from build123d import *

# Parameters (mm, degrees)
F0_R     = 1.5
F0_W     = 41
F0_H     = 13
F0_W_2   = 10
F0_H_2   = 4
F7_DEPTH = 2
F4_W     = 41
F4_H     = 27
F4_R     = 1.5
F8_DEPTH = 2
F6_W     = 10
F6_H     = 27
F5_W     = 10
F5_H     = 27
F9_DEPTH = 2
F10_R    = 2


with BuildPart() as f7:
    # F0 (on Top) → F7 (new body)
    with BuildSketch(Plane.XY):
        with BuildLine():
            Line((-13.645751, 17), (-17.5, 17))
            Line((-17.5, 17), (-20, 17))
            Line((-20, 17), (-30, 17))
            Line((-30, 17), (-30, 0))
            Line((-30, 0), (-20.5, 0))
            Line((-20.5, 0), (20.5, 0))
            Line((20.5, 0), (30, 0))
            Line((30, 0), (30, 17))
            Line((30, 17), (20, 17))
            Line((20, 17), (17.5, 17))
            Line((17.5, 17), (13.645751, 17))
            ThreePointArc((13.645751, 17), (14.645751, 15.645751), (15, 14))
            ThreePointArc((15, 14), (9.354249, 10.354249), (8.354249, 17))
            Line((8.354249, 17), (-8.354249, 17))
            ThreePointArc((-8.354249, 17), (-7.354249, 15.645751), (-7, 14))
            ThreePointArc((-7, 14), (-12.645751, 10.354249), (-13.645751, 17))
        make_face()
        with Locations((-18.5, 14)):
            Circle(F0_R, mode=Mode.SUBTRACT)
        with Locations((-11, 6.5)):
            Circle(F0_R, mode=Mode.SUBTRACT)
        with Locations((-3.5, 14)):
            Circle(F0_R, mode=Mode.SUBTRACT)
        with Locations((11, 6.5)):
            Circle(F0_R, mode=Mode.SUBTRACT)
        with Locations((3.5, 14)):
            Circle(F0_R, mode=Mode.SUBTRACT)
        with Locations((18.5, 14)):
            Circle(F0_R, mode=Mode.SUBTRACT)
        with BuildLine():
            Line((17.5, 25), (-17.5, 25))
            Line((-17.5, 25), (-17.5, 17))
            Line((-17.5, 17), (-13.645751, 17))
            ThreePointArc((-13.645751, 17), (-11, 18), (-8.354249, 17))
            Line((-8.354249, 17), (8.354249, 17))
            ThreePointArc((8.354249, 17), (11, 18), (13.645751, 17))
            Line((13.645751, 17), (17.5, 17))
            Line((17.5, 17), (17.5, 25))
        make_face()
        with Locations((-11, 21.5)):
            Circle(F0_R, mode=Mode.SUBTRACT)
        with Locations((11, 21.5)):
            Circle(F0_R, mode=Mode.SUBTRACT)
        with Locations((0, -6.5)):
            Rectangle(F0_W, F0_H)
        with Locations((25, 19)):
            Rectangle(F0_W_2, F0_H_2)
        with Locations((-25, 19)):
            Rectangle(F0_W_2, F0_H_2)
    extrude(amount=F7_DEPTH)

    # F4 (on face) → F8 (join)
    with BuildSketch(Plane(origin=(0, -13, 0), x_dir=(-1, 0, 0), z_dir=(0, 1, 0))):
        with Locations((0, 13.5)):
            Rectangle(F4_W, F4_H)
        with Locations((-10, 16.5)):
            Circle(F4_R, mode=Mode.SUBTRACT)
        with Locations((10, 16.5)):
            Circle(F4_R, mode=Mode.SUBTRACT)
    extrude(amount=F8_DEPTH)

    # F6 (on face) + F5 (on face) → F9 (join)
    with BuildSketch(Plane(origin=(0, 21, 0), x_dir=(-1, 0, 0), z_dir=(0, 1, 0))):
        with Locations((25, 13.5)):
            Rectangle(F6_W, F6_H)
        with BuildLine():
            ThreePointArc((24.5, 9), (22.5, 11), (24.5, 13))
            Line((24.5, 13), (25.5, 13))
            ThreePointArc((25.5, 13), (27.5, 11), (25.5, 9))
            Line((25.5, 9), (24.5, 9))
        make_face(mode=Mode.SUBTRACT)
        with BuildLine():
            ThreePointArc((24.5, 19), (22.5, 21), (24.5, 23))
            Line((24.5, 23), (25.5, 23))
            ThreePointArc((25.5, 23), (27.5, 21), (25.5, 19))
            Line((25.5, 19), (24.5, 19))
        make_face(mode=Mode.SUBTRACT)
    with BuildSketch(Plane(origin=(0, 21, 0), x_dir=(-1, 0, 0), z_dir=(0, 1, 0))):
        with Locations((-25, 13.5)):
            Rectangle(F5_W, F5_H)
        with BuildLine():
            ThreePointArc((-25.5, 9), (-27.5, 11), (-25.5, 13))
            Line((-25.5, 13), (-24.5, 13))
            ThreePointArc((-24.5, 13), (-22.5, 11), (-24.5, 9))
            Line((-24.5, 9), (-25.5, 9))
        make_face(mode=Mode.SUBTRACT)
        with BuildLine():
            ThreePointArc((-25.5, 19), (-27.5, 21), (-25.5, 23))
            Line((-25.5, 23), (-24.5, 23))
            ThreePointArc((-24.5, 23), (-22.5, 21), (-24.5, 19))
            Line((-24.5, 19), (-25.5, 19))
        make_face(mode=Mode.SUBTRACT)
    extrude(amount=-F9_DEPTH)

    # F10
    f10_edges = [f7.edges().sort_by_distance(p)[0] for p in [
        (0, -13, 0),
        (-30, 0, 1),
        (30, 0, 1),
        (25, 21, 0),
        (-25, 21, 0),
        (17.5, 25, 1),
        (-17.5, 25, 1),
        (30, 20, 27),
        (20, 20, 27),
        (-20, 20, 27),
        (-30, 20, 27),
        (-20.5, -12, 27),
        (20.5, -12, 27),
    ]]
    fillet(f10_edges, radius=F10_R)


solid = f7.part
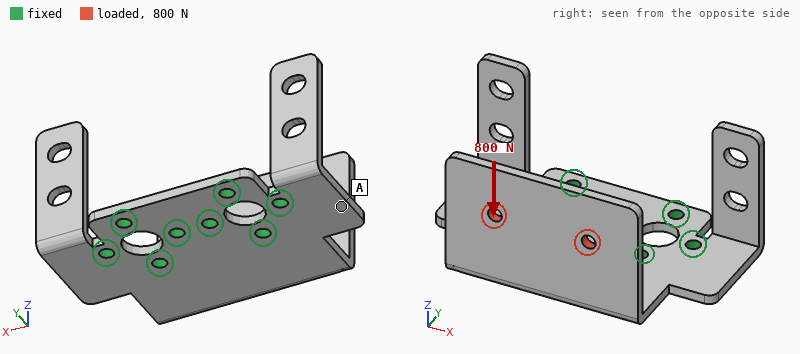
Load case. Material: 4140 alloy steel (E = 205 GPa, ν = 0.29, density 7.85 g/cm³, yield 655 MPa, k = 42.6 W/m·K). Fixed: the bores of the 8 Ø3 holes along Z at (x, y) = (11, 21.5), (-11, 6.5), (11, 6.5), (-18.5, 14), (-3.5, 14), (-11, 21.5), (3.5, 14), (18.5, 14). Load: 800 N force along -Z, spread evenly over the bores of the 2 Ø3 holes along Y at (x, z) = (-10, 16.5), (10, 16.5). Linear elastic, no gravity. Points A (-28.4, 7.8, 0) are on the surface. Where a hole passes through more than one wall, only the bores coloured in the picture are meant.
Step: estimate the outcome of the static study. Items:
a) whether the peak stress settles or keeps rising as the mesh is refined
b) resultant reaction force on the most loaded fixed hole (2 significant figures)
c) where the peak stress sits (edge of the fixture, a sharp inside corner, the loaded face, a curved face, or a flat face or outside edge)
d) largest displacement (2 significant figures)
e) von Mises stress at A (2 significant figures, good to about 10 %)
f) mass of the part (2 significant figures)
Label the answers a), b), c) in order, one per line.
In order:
a) keeps rising
b) 730 N
c) edge of the fixture
d) 0.66 mm
e) 68 MPa
f) 50 g
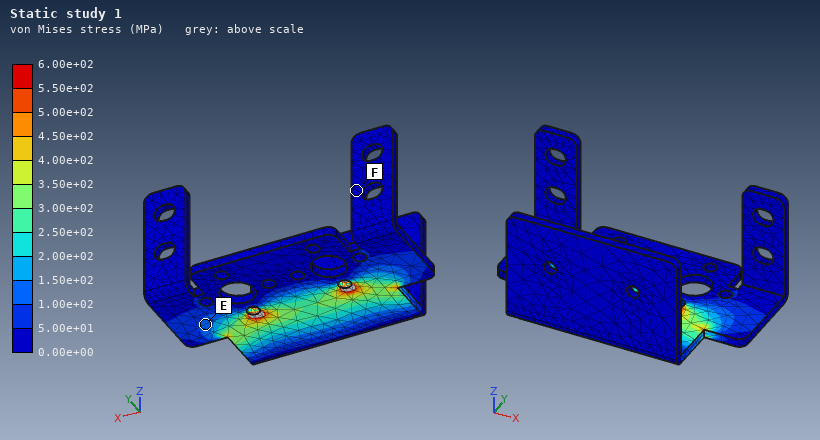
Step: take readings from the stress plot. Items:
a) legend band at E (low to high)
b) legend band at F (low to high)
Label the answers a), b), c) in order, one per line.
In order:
a) 1.00e+02 to 1.50e+02 MPa
b) 0.00e+00 to 5.00e+01 MPa
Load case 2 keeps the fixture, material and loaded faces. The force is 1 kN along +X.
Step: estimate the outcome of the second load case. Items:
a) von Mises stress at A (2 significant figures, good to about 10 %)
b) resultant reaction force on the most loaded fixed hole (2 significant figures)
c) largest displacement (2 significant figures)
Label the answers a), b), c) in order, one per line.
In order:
a) 85 MPa
b) 840 N
c) 0.43 mm
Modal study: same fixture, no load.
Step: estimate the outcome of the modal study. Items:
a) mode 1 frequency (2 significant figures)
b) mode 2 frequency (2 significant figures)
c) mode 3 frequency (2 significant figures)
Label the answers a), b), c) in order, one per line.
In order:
a) 1200 Hz
b) 1800 Hz
c) 1800 Hz
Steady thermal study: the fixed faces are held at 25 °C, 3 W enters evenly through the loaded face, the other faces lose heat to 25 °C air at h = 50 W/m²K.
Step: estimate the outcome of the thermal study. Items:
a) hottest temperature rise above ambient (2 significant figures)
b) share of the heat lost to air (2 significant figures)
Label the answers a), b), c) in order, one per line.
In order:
a) 19 K
b) 59 %
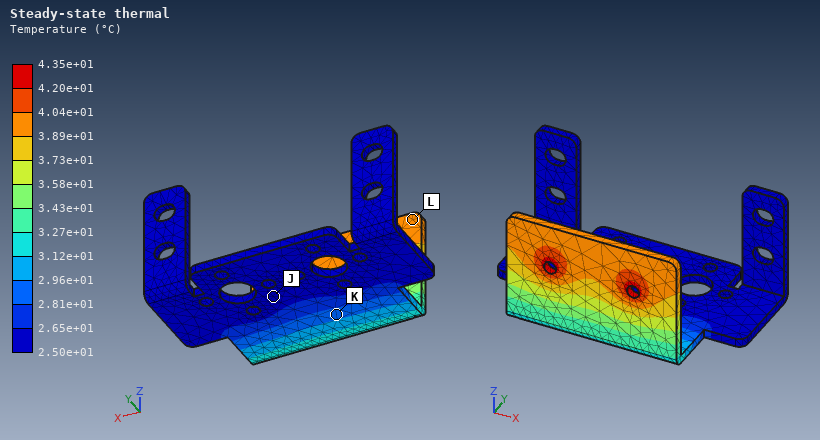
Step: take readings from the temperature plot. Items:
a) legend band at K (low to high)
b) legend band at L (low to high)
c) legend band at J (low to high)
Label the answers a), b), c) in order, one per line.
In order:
a) 2.81e+01 to 2.96e+01 °C
b) 3.89e+01 to 4.04e+01 °C
c) 2.50e+01 to 2.65e+01 °C
